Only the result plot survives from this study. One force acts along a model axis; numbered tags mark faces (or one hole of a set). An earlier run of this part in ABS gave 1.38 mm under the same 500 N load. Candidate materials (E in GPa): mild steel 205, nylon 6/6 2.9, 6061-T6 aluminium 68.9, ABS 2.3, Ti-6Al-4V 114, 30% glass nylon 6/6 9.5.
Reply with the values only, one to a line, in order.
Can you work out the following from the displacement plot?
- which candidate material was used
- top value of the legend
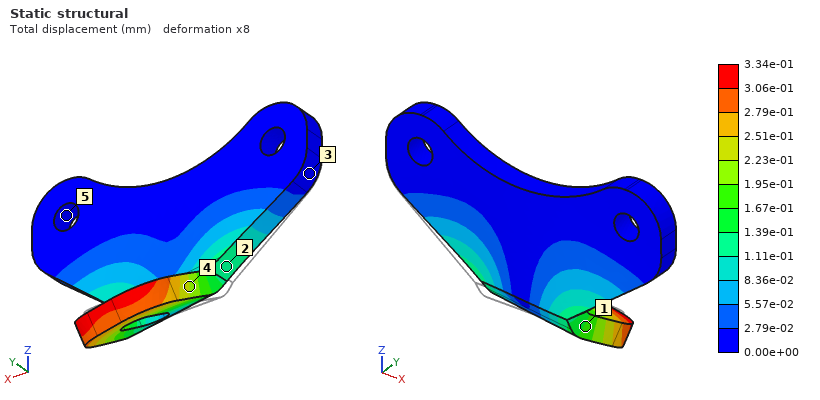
30% glass nylon 6/6
3.34e-01 mm
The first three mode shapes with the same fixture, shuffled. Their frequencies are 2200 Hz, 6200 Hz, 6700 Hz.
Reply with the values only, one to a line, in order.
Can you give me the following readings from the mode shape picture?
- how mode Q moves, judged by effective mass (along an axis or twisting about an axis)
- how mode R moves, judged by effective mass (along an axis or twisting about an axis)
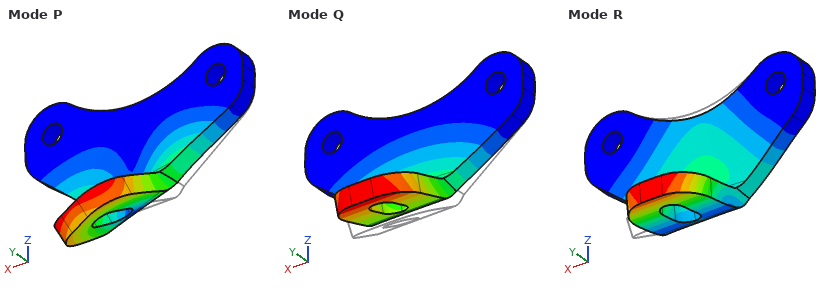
along Y
along Y
